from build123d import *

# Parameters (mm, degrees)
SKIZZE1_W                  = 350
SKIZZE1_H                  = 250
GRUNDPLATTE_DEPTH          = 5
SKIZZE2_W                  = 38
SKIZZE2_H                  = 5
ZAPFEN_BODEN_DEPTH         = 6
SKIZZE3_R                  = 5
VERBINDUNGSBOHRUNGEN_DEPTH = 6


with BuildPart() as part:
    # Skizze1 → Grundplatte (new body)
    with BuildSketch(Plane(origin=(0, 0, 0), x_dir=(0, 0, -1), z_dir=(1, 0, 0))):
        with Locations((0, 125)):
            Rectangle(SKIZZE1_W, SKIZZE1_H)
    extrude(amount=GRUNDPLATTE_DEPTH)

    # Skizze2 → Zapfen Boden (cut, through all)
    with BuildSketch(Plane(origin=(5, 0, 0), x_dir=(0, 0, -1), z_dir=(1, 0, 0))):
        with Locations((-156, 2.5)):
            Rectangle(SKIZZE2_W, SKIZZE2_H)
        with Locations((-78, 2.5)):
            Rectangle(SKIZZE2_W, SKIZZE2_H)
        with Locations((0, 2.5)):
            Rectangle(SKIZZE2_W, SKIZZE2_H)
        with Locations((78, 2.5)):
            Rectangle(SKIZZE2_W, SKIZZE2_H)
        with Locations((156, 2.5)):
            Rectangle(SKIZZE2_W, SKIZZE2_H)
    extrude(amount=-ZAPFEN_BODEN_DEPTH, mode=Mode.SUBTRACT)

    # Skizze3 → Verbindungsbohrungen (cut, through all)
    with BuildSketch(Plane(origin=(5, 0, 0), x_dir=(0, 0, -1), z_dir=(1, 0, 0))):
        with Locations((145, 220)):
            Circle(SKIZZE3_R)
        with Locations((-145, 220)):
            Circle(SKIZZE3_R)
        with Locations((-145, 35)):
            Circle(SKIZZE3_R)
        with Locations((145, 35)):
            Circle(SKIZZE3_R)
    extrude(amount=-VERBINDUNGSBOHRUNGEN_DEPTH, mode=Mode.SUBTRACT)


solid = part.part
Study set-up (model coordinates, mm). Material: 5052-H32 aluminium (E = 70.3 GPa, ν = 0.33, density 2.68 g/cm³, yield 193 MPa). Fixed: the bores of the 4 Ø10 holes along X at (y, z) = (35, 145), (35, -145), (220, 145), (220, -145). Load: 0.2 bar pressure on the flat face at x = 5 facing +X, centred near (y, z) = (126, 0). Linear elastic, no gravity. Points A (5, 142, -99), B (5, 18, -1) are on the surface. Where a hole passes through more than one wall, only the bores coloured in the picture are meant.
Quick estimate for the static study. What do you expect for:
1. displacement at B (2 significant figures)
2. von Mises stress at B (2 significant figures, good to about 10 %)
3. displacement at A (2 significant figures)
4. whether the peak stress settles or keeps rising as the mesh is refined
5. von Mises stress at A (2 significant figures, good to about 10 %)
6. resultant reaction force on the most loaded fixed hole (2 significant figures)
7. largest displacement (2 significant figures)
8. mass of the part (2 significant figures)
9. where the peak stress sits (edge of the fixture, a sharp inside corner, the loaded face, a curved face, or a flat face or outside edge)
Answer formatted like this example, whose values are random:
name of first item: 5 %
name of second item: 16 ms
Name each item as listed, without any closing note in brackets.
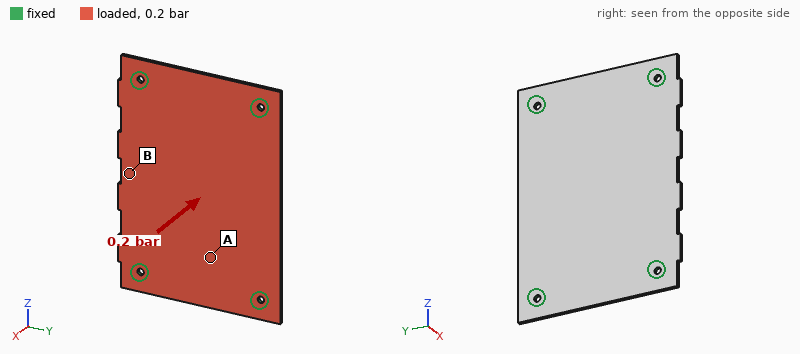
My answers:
displacement at B: 0.62 mm
von Mises stress at B: 21 MPa
displacement at A: 0.34 mm
whether the peak stress settles or keeps rising as the mesh is refined: keeps rising
von Mises stress at A: 8.7 MPa
resultant reaction force on the most loaded fixed hole: 440 N
largest displacement: 0.69 mm
mass of the part: 1.2 kg
where the peak stress sits: edge of the fixture
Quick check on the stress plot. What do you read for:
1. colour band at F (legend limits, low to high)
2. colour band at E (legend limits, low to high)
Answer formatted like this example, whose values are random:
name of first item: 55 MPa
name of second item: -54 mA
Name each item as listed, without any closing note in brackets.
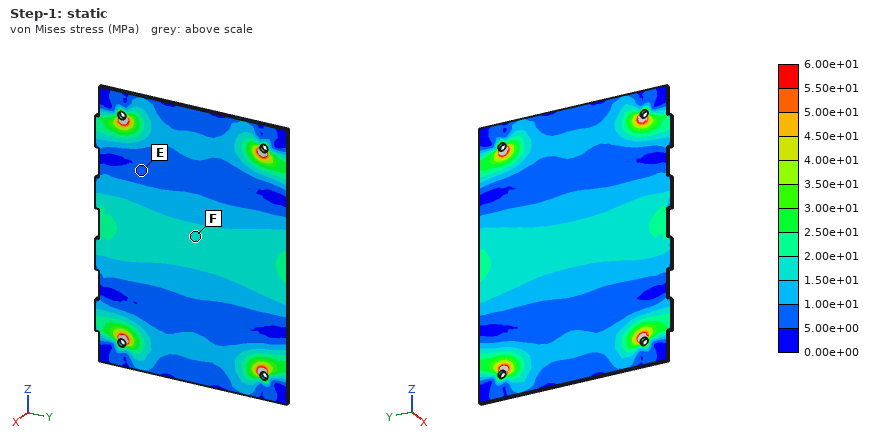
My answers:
colour band at F: 1.50e+01 to 2.00e+01 MPa
colour band at E: 5.00e+00 to 1.00e+01 MPa
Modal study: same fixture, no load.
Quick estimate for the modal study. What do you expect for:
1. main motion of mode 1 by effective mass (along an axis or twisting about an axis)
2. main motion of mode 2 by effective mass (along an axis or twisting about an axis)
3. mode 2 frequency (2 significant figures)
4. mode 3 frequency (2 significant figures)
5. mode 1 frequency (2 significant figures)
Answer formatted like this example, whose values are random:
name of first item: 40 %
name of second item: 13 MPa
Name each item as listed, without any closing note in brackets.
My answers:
main motion of mode 1 by effective mass: along X
main motion of mode 2 by effective mass: twisting about Z
mode 2 frequency: 390 Hz
mode 3 frequency: 630 Hz
mode 1 frequency: 270 Hz
